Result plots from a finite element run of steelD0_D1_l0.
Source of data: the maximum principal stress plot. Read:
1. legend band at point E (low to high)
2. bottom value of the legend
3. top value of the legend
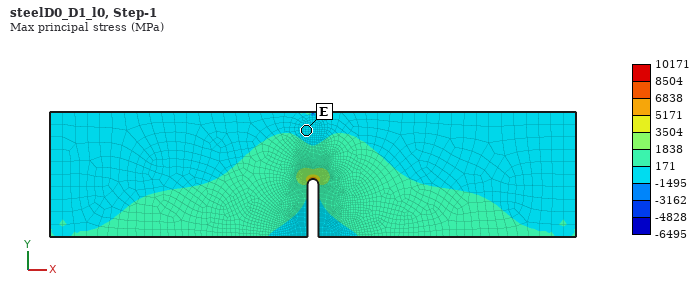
-1495 to 171 MPa
-6495 MPa
10171 MPa
